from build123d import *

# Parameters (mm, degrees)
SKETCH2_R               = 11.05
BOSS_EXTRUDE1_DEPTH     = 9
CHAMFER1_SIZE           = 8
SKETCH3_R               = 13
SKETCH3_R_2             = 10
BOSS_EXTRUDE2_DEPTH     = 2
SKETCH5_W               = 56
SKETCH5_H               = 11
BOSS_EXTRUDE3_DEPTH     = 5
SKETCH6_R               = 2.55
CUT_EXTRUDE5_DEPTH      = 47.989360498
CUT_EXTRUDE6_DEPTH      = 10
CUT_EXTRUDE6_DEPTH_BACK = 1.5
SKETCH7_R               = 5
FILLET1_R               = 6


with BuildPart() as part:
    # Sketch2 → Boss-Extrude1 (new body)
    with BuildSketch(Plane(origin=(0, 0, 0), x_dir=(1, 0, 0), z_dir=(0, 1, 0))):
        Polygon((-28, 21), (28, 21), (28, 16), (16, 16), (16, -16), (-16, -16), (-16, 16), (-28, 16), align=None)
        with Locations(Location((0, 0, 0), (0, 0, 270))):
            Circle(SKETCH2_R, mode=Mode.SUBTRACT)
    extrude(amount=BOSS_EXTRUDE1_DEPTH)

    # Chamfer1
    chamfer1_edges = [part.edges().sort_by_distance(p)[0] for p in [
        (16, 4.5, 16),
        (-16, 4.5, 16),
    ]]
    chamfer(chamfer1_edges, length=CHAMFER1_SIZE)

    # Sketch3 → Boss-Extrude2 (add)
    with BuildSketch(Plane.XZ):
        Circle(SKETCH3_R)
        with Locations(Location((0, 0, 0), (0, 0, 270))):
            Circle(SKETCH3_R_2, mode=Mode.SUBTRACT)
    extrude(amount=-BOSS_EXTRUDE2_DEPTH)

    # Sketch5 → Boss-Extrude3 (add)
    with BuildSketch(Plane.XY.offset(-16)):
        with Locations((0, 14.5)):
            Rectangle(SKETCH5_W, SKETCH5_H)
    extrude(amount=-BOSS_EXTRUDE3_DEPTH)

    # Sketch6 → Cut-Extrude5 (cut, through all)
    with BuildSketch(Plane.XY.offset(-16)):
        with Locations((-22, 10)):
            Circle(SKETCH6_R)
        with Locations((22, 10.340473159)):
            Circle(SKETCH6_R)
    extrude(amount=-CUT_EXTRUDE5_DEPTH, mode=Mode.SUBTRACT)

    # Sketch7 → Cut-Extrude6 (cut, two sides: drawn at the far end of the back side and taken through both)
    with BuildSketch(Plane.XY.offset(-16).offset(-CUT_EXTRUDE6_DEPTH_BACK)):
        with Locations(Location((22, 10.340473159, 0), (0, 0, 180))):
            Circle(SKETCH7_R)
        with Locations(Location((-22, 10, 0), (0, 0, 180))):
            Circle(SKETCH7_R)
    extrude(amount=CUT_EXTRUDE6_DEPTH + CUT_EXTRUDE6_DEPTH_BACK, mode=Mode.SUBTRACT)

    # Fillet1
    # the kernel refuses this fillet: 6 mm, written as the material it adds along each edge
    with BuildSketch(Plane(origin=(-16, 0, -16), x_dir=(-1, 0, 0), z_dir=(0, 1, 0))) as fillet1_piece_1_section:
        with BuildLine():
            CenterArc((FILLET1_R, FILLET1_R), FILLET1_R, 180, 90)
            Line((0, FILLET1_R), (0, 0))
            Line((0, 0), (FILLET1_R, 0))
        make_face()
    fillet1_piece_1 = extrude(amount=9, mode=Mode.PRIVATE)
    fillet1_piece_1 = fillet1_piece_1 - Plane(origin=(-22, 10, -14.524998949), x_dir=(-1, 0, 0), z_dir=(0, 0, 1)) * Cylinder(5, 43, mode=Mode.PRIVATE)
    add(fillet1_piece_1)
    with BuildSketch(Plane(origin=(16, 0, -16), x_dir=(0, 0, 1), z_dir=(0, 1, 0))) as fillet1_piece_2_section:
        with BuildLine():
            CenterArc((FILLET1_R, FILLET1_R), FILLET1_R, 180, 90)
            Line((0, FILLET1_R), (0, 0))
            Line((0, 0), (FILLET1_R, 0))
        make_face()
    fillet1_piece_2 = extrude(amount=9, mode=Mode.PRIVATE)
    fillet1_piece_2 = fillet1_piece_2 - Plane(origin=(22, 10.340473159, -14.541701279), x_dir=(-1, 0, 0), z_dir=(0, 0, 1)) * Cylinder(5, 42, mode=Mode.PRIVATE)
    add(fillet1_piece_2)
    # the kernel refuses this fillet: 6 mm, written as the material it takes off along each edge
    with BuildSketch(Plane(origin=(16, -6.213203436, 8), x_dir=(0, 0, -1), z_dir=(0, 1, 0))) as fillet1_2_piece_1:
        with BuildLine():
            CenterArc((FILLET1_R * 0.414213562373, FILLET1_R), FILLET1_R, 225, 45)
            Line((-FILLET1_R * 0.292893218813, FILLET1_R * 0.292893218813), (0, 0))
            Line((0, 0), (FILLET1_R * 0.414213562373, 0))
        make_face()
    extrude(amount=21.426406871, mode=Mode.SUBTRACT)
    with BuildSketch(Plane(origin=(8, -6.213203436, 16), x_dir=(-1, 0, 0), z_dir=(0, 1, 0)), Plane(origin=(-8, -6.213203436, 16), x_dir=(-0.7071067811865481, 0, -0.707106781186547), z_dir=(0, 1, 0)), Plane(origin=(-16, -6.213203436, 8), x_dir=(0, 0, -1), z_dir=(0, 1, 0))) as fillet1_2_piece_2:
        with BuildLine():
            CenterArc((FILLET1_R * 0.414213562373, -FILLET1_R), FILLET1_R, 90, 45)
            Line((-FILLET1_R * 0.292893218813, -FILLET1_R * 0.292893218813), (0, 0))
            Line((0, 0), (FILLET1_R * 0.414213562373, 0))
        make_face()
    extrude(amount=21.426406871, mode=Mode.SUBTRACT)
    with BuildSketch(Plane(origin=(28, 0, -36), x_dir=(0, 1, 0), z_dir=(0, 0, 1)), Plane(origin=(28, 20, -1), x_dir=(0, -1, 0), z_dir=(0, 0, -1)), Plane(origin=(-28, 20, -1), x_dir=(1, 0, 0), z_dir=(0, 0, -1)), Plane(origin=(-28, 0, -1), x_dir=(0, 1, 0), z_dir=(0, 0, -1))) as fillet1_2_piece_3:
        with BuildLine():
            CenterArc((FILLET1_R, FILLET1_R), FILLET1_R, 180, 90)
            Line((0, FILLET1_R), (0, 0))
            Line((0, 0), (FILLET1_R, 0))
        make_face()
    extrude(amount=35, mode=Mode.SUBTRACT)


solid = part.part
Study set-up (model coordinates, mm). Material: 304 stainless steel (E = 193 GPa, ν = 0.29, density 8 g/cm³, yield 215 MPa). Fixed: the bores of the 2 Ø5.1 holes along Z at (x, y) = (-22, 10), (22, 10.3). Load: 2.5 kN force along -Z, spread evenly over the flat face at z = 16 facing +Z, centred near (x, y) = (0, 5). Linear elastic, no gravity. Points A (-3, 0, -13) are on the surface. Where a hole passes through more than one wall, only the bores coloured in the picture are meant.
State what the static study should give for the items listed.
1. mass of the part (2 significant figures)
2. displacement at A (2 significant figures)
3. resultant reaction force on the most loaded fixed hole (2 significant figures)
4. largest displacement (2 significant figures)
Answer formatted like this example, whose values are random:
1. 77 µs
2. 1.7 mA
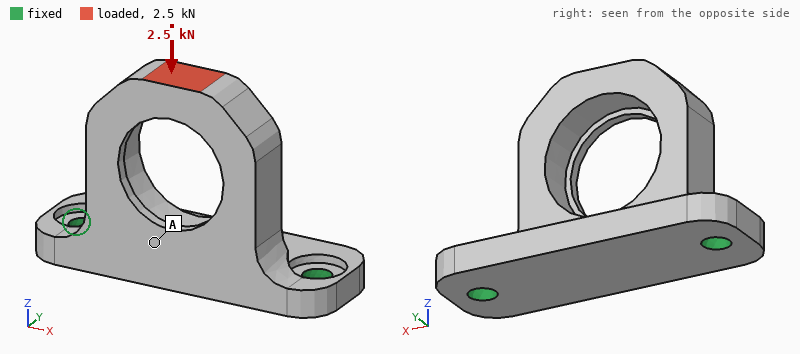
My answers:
1. 84 g
2. 14 µm
3. 1.4 kN
4. 43 µm
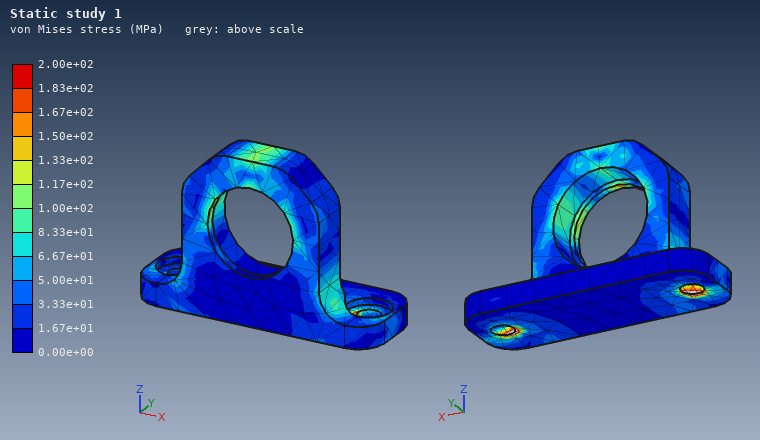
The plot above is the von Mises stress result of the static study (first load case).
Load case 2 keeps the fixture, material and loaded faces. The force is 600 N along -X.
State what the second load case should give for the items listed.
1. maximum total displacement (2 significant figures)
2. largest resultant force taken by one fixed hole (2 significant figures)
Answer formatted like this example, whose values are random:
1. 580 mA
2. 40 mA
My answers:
1. 15 µm
2. 620 N
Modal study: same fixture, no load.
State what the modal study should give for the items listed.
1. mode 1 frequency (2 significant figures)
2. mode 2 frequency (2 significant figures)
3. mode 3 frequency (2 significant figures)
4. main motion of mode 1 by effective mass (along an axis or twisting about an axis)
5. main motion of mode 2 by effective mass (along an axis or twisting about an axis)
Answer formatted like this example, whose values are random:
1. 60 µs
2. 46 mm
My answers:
1. 3000 Hz
2. 8100 Hz
3. 11 kHz
4. along Y
5. along X
